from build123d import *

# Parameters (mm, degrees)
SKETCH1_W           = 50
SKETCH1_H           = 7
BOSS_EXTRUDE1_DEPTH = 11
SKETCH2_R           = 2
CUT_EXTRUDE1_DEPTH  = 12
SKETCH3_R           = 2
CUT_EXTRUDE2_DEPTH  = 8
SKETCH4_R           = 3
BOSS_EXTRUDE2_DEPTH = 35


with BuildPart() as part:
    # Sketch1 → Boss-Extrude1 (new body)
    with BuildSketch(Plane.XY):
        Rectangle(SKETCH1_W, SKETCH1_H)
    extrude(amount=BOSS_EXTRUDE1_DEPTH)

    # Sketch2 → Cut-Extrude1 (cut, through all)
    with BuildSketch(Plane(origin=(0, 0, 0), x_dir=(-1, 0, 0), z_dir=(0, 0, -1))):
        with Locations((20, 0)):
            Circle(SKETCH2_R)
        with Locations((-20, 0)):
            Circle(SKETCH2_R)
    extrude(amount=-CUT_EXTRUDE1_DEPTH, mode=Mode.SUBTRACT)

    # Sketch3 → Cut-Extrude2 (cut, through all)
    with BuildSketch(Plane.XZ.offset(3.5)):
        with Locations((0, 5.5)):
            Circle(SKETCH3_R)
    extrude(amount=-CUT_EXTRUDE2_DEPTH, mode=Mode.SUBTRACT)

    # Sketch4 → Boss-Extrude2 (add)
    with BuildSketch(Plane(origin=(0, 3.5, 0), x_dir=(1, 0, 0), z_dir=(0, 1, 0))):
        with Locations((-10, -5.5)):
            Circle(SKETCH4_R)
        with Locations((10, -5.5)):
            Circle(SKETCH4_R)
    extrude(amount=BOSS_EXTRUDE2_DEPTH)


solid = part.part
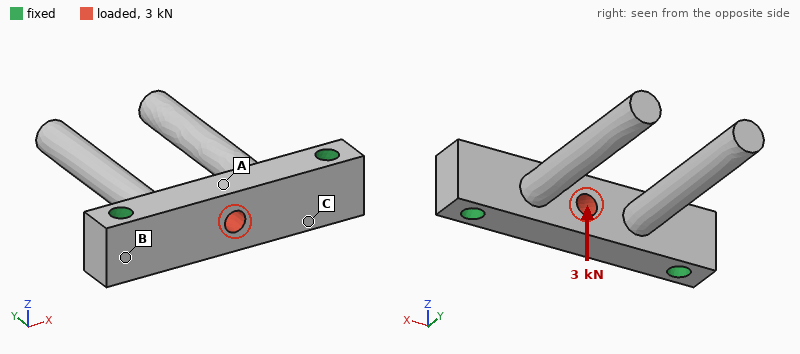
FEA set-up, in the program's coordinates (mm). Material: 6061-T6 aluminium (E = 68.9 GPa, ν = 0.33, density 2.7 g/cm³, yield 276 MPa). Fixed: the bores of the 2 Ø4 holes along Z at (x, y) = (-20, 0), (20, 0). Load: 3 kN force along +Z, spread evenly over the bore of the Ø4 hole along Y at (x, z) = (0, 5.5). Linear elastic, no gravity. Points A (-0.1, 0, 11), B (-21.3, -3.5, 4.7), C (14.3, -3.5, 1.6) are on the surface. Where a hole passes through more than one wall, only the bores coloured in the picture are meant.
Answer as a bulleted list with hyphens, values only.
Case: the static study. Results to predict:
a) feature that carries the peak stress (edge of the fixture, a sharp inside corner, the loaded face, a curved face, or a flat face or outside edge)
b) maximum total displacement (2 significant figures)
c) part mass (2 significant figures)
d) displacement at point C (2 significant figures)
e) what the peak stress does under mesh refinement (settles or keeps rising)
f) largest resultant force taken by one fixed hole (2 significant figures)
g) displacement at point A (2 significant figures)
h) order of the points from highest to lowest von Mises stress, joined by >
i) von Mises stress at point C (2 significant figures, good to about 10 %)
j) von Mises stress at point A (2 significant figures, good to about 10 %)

- edge of the fixture
- 32 µm
- 15 g
- 6.7 µm
- keeps rising
- 1.5 kN
- 29 µm
- A > C > B
- 42 MPa
- 100 MPa
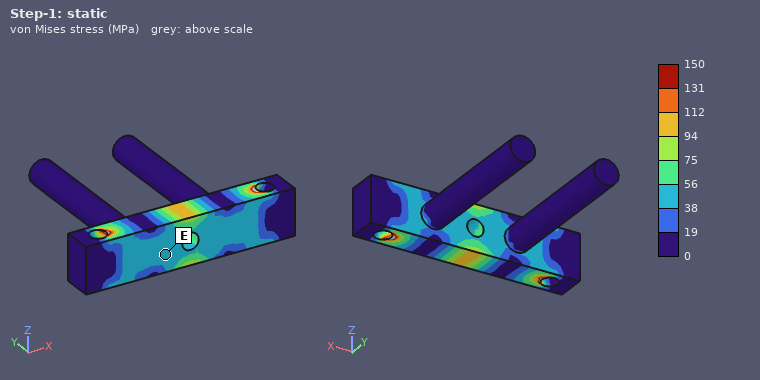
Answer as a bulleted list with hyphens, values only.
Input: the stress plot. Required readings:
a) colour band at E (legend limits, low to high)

- 38 to 56 MPa
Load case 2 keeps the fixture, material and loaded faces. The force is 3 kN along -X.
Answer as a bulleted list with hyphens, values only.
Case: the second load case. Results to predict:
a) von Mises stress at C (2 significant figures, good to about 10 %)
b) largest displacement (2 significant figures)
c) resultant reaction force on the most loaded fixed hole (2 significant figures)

- 17 MPa
- 5.8 µm
- 1.5 kN
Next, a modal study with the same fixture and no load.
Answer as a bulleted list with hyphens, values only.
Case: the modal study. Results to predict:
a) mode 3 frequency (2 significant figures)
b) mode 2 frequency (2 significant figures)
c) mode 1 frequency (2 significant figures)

- 3000 Hz
- 3000 Hz
- 2900 Hz
